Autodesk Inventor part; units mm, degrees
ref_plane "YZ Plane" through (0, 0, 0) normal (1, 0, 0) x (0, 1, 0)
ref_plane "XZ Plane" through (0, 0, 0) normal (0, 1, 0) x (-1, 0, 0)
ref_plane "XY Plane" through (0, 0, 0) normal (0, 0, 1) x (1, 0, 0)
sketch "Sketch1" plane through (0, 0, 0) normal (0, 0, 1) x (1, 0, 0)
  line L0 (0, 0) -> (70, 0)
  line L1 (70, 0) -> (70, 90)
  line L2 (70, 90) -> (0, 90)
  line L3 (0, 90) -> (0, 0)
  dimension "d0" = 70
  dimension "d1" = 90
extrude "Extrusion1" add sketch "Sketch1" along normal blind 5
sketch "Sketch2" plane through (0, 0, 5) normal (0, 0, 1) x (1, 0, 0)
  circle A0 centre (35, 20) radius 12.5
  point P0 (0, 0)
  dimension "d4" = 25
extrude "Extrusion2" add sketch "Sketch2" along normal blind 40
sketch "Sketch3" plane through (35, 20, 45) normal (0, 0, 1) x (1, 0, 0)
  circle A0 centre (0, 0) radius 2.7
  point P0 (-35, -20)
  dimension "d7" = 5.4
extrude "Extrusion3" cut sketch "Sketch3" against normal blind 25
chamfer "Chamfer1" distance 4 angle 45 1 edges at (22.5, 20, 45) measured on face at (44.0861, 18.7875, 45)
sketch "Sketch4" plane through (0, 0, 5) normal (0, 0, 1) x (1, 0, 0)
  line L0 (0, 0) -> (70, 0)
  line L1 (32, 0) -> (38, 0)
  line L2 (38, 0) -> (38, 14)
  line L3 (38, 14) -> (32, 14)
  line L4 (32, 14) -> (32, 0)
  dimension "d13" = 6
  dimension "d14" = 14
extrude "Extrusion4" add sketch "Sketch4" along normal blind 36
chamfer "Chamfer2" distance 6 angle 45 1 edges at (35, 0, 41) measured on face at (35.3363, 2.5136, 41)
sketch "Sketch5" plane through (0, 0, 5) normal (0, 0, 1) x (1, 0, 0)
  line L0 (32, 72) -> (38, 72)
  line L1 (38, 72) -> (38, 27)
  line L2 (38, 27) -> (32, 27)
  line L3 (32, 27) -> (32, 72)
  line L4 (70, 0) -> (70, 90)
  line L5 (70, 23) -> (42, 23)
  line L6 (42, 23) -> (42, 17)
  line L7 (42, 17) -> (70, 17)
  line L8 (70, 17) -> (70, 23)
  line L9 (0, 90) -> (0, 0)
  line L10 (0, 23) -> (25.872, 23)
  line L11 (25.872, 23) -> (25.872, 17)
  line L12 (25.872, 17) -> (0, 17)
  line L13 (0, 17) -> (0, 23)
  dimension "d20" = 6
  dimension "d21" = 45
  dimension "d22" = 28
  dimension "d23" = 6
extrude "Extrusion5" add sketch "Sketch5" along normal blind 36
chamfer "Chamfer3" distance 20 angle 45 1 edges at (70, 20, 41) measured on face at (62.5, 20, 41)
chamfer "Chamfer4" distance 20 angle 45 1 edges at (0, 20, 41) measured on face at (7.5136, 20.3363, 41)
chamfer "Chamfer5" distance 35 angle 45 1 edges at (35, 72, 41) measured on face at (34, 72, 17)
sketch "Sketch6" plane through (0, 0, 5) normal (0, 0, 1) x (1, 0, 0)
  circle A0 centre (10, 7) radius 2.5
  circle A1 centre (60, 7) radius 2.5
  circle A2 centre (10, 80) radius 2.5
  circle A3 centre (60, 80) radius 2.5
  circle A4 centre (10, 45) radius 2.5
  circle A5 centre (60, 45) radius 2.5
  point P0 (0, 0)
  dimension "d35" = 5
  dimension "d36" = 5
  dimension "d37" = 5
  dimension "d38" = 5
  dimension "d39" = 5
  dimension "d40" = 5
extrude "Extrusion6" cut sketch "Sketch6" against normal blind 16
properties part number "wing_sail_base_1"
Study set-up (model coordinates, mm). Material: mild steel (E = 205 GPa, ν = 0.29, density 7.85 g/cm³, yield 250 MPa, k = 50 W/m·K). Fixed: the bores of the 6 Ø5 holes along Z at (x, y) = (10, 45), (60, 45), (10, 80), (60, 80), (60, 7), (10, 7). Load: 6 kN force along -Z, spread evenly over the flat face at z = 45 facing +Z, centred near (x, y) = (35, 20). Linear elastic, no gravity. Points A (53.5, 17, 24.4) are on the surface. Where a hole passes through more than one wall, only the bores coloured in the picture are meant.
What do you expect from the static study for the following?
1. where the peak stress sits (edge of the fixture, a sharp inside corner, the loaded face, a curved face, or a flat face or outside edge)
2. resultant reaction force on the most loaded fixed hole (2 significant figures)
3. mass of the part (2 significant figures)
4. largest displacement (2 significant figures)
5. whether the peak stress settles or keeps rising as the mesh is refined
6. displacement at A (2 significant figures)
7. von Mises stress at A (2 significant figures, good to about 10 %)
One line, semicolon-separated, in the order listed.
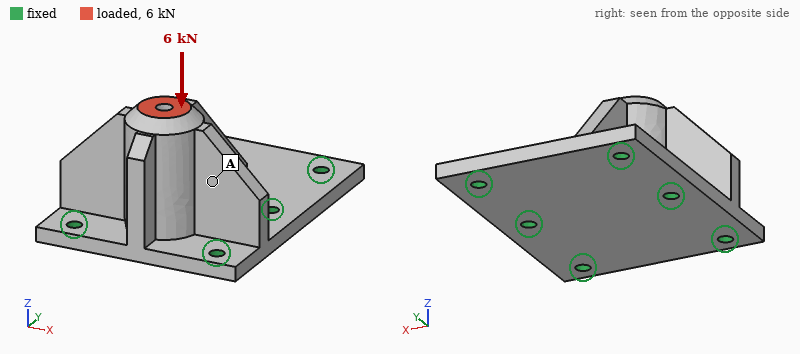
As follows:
edge of the fixture; 2.2 kN; 500 g; 16 µm; keeps rising; 11 µm; 16 MPa
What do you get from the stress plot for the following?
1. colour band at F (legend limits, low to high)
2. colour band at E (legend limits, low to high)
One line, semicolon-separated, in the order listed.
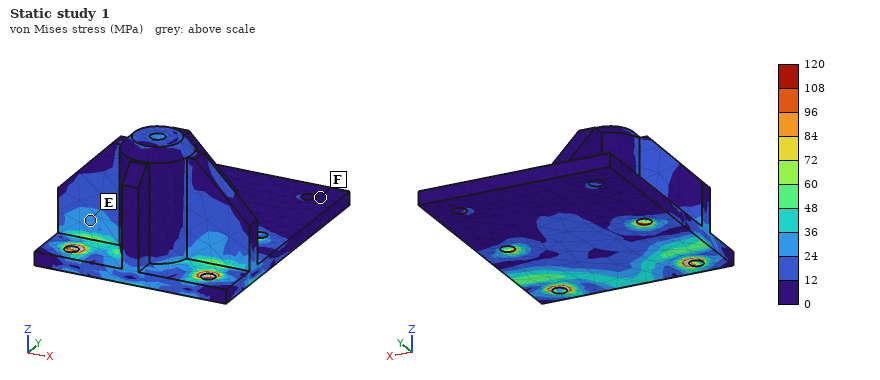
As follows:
0 to 12 MPa; 24 to 36 MPa
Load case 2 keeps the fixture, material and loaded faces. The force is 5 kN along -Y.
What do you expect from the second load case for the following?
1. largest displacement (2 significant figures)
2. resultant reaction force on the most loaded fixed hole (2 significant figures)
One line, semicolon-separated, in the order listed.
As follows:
54 µm; 2.3 kN
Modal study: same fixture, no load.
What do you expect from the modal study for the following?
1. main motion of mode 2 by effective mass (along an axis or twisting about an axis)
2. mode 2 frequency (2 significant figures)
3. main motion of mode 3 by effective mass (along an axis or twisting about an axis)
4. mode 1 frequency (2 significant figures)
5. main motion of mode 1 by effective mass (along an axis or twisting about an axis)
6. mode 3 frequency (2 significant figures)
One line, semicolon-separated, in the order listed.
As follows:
along X; 6200 Hz; along Z; 5200 Hz; along Y; 6700 Hz
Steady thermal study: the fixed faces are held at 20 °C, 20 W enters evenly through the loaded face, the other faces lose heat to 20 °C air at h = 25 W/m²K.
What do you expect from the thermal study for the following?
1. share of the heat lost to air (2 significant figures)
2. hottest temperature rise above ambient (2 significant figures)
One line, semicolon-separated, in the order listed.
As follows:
22 %; 36 K
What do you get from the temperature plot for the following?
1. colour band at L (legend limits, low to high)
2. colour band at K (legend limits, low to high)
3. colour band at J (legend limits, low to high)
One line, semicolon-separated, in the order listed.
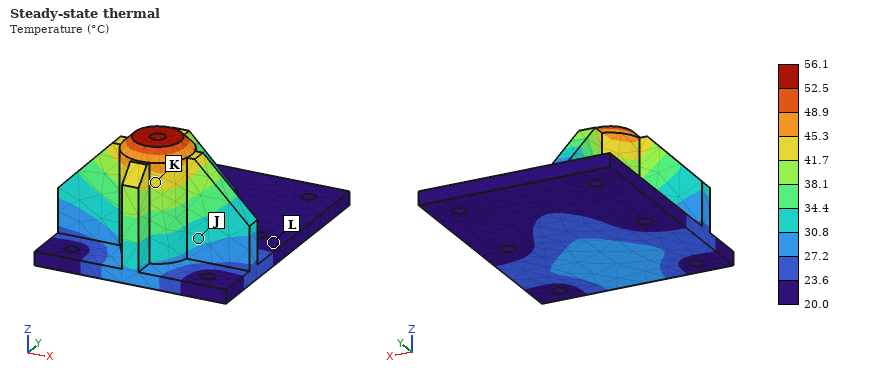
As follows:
20.0 to 23.6 °C; 41.7 to 45.3 °C; 30.8 to 34.4 °C
